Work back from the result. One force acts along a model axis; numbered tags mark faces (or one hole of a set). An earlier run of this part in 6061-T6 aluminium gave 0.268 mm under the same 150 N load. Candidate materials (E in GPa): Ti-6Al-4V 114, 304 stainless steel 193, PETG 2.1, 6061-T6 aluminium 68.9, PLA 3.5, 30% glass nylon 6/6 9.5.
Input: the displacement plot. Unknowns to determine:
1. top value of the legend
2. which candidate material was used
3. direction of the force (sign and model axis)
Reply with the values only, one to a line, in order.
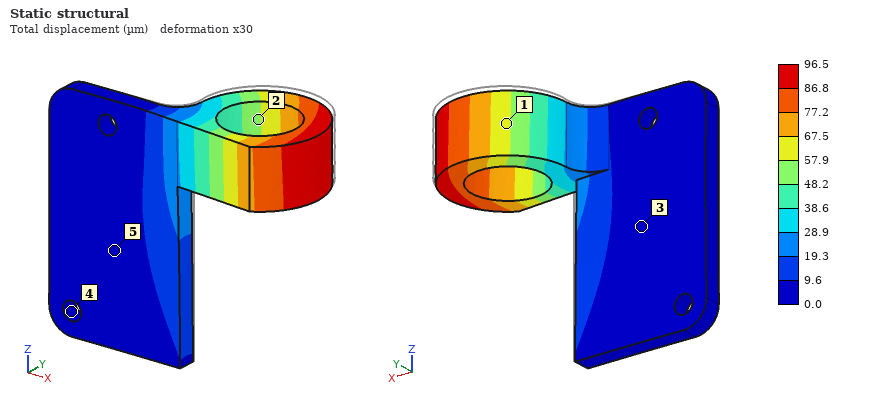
96.5 µm
304 stainless steel
-Y
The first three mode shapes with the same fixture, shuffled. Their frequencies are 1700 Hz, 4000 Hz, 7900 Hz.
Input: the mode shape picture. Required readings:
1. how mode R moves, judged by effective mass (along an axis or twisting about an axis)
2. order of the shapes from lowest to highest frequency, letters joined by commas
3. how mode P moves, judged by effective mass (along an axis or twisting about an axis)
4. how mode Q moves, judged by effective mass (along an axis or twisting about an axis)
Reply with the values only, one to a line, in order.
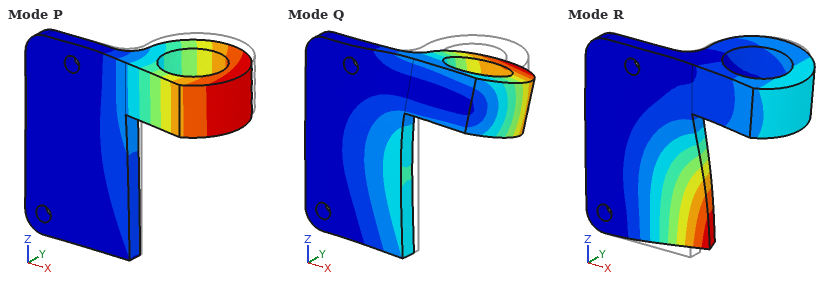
along Y
P, Q, R
along Y
along Z
